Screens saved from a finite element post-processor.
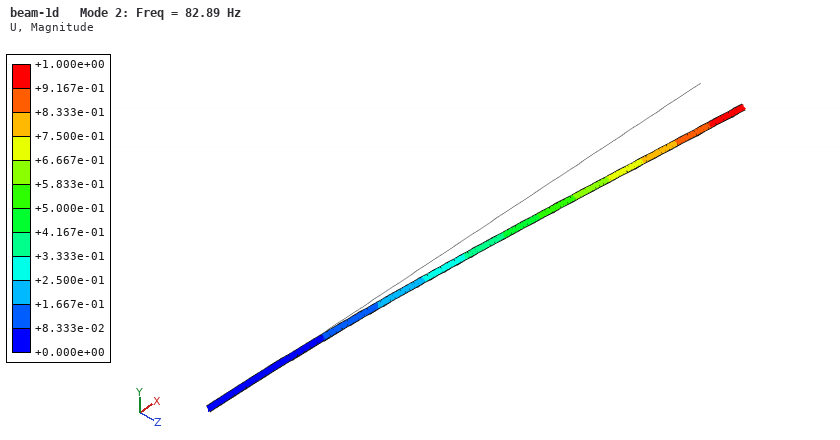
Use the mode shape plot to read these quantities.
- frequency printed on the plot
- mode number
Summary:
82.89 Hz
2
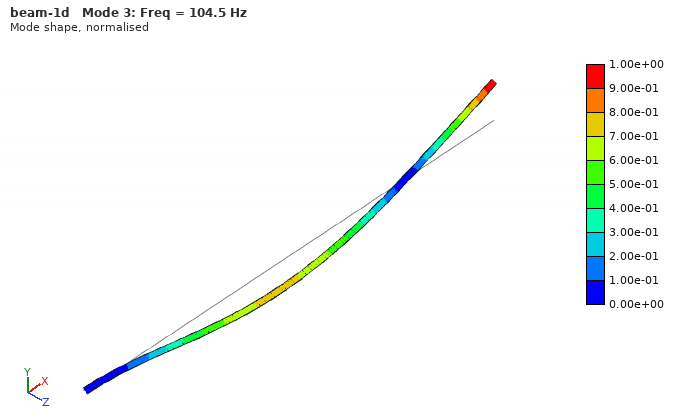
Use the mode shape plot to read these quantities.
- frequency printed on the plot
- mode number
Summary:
104.5 Hz
3
